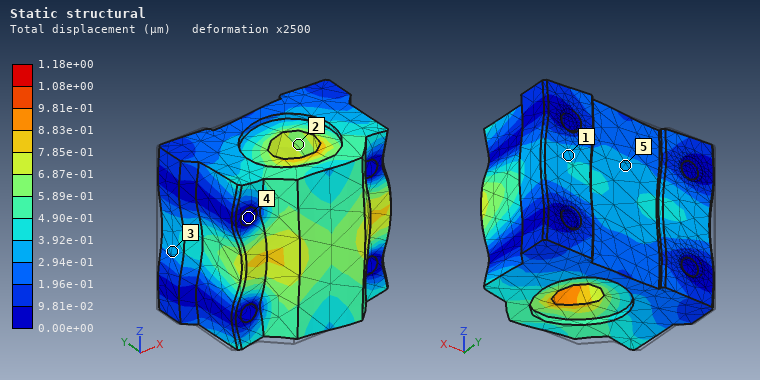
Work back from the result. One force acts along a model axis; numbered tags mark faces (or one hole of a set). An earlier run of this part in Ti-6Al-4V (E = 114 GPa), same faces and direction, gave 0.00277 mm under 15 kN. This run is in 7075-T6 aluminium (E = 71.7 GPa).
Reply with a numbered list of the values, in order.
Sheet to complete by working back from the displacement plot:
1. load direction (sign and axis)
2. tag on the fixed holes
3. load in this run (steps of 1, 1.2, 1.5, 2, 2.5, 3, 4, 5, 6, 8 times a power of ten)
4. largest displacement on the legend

1. +X
2. 4
3. 4 kN
4. 1.18e+00 µm
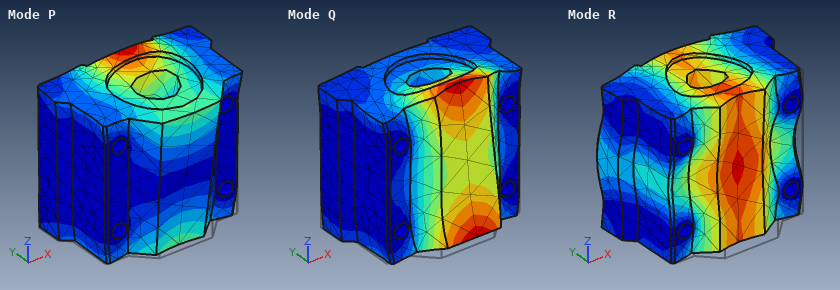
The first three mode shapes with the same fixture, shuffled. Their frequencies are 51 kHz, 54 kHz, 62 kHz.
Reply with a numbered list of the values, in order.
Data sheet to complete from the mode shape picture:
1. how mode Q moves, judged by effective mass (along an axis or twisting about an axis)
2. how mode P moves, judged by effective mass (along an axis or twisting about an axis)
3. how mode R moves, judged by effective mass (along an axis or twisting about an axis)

1. along Z
2. along Z
3. along Y
